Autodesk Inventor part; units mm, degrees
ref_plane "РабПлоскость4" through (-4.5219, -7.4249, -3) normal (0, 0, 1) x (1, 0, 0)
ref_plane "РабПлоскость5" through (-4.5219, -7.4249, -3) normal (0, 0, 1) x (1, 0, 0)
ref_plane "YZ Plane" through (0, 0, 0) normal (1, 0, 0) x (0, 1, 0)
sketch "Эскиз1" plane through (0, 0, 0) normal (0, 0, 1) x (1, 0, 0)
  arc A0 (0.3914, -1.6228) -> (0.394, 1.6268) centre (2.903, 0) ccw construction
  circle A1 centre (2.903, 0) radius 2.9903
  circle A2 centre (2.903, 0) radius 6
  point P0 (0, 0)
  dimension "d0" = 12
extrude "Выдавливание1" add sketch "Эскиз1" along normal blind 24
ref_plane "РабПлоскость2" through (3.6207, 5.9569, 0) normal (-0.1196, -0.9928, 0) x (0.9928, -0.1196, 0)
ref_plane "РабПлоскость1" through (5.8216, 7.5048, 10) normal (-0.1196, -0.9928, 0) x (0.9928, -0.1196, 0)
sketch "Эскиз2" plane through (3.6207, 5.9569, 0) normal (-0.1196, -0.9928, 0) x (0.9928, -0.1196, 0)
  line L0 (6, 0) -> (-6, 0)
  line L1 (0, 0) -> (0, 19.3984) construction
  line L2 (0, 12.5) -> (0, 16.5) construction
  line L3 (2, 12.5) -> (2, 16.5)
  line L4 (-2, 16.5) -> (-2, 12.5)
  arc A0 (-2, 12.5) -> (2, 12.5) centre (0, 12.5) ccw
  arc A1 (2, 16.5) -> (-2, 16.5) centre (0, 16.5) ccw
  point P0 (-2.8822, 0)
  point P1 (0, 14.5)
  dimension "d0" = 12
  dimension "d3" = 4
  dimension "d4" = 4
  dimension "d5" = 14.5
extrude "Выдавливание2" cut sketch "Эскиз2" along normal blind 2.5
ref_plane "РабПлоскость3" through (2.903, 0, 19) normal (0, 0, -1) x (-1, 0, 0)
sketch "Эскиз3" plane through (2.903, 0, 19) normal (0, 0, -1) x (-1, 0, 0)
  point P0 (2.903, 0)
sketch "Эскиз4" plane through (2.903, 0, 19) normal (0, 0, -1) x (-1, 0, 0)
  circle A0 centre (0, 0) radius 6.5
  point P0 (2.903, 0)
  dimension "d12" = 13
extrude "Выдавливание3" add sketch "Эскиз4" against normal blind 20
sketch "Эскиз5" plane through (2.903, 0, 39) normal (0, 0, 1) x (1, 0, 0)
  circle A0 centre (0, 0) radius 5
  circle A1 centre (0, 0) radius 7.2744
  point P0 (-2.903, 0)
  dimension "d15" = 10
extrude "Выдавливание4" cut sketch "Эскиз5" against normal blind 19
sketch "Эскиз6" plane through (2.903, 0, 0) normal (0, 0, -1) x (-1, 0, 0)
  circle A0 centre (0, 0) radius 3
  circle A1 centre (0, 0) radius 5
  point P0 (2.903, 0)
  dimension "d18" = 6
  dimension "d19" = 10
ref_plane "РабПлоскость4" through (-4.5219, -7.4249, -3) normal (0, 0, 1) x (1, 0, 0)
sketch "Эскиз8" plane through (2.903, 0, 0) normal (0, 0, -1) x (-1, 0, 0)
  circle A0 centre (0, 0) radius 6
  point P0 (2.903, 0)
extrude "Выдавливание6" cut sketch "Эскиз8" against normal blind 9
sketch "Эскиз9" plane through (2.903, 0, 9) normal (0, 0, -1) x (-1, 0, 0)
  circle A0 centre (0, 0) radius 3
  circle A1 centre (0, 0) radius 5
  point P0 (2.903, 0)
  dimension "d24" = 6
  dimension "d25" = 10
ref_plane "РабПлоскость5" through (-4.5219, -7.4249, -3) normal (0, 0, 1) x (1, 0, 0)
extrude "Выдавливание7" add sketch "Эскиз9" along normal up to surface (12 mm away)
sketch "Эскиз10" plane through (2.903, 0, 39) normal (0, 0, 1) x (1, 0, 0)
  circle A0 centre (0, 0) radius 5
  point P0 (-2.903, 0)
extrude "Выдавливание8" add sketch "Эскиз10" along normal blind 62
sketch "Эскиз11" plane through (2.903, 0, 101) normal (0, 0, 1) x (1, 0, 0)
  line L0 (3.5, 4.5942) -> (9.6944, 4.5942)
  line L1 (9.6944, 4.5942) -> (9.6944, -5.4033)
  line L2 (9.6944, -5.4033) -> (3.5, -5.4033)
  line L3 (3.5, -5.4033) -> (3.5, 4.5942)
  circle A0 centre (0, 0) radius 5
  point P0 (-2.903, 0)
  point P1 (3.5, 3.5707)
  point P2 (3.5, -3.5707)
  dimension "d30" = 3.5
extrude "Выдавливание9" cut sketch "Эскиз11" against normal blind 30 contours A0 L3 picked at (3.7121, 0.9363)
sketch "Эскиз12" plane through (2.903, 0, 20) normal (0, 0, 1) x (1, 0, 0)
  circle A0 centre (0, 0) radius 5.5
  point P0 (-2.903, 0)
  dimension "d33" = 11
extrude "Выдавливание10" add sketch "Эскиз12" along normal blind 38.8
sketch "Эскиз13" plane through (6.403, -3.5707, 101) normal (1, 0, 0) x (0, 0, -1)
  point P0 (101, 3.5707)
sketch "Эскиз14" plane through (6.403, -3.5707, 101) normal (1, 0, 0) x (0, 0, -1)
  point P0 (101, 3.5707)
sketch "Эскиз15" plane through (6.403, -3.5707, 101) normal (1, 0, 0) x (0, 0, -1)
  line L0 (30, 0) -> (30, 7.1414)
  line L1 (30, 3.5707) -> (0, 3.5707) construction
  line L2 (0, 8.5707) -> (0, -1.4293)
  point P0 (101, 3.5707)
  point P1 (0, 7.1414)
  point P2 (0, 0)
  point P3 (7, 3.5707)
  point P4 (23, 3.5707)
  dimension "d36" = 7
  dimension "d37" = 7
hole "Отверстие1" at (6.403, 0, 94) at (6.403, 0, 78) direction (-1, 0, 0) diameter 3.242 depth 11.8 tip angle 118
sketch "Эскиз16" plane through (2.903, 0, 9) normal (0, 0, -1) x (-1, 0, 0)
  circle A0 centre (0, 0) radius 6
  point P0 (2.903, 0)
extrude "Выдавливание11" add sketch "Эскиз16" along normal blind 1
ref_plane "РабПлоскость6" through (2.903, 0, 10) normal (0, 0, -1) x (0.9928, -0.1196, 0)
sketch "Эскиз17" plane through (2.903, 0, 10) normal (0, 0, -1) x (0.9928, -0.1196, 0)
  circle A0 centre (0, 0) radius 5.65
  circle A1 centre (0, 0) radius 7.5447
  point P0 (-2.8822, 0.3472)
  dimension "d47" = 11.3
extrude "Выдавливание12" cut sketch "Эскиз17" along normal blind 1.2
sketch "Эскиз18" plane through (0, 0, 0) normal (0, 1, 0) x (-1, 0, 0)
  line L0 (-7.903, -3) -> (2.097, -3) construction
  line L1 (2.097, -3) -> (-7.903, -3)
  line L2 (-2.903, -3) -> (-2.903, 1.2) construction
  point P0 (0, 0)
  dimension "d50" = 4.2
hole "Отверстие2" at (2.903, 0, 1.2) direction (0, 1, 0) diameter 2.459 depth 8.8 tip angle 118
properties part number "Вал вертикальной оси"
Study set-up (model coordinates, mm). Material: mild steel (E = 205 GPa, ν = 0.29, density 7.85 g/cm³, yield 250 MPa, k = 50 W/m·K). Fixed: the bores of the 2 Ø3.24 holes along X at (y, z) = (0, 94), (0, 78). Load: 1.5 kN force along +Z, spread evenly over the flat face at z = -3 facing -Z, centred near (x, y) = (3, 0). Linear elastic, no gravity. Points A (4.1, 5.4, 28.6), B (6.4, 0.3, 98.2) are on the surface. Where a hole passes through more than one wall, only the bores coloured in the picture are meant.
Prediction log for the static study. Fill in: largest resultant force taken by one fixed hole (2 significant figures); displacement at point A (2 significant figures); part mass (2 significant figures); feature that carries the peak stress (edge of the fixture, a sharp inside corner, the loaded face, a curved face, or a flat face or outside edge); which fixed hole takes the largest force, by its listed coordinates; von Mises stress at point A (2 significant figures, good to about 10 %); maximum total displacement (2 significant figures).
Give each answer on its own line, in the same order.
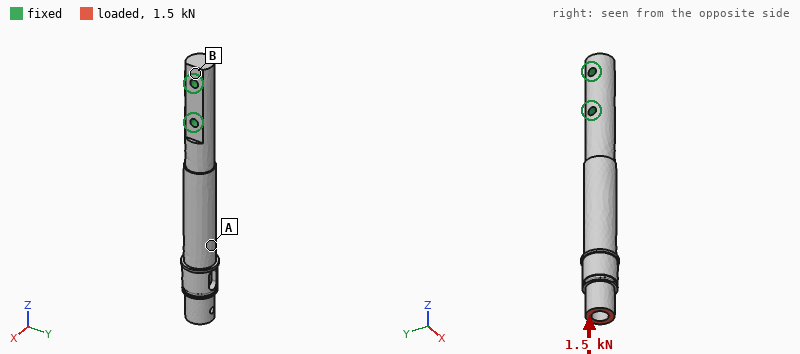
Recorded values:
1.4 kN
5.6 µm
64 g
a curved face
(0, 78)
15 MPa
11 µm
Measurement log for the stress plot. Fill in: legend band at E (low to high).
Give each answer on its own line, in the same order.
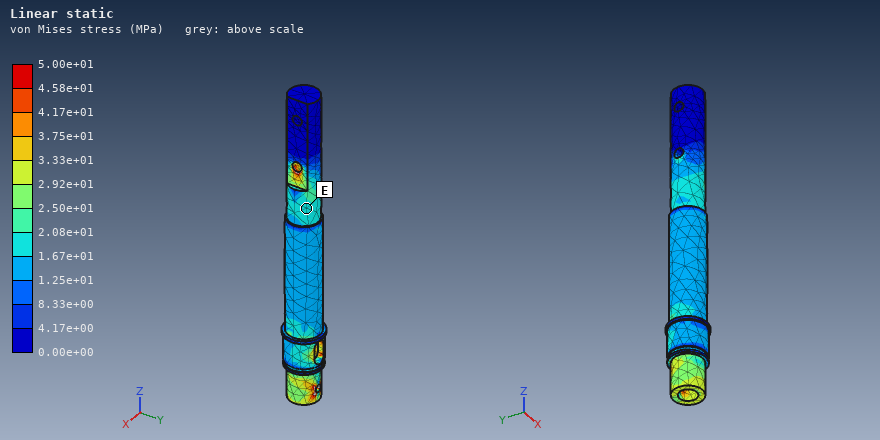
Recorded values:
1.67e+01 to 2.08e+01 MPa
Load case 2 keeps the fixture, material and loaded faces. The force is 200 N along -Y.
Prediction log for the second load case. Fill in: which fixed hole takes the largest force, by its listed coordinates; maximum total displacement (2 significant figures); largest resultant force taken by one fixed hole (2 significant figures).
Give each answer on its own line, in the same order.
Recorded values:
(0, 78)
0.34 mm
610 N
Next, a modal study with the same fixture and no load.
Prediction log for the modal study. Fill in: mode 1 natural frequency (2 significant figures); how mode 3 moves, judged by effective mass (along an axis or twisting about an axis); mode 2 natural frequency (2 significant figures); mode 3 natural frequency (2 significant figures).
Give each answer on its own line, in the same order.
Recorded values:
1100 Hz
along Y
1100 Hz
7000 Hz
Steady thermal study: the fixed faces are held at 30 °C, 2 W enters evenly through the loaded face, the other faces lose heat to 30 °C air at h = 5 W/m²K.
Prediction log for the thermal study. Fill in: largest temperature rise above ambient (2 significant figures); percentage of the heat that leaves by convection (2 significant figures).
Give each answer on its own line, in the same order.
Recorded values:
38 K
16 %
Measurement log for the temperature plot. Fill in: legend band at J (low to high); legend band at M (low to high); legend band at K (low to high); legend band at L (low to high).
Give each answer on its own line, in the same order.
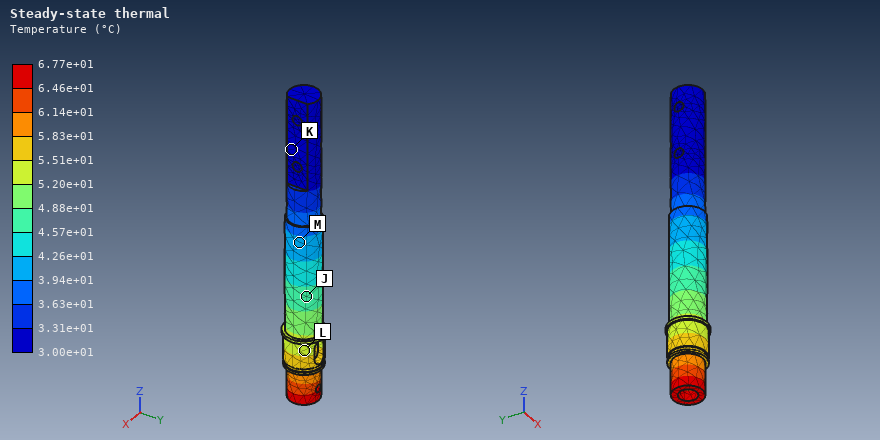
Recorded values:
4.57e+01 to 4.88e+01 °C
3.94e+01 to 4.26e+01 °C
3.00e+01 to 3.31e+01 °C
5.20e+01 to 5.51e+01 °C
